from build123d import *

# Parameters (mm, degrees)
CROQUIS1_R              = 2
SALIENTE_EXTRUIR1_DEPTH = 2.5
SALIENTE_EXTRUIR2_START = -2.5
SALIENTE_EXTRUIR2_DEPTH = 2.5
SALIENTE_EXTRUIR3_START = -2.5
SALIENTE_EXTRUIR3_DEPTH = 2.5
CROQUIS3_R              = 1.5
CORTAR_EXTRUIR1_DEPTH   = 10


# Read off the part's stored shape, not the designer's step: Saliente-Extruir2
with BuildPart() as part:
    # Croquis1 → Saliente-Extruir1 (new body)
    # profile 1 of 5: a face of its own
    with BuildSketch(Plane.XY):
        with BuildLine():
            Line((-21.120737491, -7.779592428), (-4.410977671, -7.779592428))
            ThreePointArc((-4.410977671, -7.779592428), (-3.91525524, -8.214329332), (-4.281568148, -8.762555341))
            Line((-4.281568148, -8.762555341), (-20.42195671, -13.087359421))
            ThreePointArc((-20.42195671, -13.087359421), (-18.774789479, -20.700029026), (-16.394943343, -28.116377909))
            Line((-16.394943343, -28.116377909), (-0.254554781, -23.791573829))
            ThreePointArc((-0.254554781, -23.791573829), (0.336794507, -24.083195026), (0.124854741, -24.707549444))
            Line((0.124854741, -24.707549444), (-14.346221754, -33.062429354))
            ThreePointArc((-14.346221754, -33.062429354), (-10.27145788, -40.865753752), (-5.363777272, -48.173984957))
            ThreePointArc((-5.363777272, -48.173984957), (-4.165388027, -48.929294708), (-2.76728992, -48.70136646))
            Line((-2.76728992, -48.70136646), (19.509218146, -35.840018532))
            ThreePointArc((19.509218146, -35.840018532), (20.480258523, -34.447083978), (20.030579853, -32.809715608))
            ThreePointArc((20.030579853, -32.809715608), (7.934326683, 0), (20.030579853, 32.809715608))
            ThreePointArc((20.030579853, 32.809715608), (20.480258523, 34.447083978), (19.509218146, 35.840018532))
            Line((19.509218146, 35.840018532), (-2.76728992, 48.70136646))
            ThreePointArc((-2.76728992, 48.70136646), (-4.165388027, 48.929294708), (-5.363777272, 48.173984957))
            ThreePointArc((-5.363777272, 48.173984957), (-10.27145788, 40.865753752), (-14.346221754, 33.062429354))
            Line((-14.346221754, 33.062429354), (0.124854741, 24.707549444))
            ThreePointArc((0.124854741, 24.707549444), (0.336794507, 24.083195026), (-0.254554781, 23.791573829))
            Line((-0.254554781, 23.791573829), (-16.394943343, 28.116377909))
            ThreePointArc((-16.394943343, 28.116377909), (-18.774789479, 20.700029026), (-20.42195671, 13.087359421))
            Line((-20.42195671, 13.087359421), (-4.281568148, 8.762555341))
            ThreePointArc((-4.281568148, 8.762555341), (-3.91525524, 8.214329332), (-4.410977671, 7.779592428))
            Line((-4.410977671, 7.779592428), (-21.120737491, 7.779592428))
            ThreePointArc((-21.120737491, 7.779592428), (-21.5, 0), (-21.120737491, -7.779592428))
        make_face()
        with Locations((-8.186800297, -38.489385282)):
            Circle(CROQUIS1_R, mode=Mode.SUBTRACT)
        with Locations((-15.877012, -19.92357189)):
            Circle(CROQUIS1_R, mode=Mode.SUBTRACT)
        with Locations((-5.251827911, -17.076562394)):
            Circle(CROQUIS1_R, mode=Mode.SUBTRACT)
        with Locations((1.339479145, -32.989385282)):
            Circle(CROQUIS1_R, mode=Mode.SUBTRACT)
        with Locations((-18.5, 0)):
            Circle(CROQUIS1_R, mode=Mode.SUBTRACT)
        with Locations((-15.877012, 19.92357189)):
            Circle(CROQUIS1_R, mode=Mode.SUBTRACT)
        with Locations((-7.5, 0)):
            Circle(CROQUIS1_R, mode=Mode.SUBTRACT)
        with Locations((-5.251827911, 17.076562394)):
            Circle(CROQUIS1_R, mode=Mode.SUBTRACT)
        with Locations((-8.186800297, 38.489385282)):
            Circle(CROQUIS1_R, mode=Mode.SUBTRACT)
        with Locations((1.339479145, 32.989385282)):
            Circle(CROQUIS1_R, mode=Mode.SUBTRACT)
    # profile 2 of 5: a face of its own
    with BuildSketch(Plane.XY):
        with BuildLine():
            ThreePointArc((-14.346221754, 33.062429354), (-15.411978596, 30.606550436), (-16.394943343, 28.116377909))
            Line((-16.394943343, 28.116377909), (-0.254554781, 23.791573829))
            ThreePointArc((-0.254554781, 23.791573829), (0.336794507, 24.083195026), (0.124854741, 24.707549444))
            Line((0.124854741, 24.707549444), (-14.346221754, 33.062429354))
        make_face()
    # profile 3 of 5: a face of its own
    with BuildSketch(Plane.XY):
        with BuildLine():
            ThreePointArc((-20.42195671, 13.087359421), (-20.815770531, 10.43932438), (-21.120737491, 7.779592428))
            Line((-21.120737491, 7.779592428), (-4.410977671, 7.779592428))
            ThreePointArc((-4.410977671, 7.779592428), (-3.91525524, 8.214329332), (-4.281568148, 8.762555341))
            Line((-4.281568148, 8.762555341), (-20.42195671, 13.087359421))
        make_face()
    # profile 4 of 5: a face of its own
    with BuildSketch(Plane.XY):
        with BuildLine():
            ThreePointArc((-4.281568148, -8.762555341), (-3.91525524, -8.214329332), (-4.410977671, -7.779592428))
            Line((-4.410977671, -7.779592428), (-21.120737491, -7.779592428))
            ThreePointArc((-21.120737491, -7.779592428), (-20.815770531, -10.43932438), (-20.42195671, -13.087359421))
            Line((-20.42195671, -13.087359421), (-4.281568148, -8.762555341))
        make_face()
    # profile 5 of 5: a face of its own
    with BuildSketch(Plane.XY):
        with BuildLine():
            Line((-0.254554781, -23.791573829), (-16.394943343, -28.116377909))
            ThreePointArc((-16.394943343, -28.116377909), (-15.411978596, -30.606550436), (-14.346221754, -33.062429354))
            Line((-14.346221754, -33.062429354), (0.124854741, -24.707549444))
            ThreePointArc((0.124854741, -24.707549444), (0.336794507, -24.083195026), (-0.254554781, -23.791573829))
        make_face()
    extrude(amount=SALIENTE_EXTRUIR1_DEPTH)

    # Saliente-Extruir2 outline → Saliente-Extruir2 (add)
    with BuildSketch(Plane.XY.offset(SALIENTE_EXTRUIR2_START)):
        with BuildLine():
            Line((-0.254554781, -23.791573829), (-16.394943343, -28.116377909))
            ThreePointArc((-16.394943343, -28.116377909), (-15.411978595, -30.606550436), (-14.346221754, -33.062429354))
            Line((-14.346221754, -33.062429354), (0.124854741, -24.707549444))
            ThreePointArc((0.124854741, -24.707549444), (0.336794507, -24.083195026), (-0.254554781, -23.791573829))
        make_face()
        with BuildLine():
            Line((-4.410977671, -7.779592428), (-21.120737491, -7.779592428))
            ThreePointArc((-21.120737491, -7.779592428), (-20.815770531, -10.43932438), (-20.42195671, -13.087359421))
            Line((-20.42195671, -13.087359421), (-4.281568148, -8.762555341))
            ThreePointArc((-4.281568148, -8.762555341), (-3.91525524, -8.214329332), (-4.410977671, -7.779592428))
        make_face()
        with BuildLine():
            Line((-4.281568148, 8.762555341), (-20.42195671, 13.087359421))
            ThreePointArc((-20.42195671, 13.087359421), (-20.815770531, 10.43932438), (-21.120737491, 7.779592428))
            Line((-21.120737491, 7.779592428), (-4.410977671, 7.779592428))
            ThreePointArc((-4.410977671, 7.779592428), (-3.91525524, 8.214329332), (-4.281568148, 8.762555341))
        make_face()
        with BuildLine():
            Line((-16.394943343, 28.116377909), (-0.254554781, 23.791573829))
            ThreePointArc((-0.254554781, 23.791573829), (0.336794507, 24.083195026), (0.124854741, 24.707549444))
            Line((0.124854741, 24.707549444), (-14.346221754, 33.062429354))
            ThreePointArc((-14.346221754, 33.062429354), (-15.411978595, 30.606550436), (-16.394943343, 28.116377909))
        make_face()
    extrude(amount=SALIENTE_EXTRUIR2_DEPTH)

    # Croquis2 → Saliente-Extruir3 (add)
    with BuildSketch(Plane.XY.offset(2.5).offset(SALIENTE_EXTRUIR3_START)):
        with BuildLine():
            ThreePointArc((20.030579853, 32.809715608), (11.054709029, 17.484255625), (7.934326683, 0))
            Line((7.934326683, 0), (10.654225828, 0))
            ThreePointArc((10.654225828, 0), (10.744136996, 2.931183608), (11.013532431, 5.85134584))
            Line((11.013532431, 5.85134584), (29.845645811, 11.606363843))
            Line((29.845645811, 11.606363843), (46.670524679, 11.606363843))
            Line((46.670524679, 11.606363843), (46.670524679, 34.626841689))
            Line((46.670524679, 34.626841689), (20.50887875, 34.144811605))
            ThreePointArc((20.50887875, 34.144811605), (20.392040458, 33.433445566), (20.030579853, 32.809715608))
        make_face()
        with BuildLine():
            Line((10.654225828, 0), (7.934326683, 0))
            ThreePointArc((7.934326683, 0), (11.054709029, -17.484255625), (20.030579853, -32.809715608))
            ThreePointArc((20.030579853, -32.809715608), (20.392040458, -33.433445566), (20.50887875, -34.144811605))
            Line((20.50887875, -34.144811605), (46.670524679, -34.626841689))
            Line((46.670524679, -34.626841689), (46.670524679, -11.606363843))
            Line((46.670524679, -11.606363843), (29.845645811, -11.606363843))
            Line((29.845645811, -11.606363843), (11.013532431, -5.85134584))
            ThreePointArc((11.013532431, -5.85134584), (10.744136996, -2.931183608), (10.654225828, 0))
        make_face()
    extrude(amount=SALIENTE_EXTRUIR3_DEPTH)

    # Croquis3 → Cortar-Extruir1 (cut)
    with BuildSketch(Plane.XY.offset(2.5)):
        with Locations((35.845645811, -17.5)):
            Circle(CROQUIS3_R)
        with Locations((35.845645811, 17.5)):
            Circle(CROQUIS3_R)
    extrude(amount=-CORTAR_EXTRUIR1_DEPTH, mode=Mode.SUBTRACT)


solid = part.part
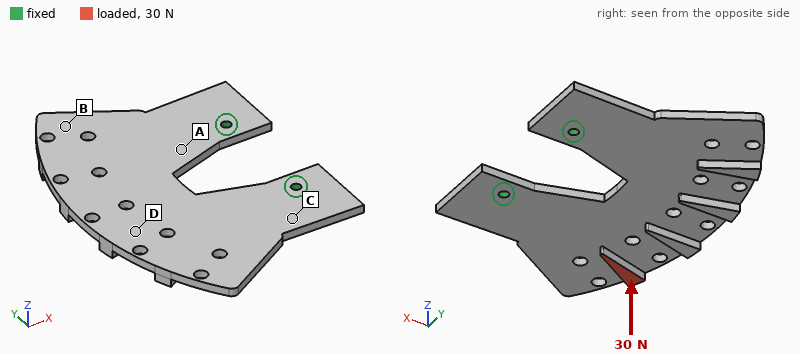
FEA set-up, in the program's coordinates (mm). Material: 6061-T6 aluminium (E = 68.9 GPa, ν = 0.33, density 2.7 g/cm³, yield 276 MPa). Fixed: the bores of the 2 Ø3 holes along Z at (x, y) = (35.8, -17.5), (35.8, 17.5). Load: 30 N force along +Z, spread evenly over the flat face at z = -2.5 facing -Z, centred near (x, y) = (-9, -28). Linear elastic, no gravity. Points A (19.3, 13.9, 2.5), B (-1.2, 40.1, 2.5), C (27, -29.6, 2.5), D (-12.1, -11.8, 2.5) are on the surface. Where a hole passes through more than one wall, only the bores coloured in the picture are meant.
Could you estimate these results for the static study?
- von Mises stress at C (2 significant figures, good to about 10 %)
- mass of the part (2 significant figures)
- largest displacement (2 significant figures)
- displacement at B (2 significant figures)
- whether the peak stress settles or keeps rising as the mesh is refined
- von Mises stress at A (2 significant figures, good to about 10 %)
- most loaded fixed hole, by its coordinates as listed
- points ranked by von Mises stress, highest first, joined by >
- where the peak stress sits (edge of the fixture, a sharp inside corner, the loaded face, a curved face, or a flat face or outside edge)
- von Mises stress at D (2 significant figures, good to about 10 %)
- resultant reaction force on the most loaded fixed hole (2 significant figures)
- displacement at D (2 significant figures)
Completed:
26 MPa
30 g
0.37 mm
0.081 mm
keeps rising
14 MPa
(35.8, -17.5)
C > A > D > B
edge of the fixture
6.9 MPa
27 N
0.28 mm
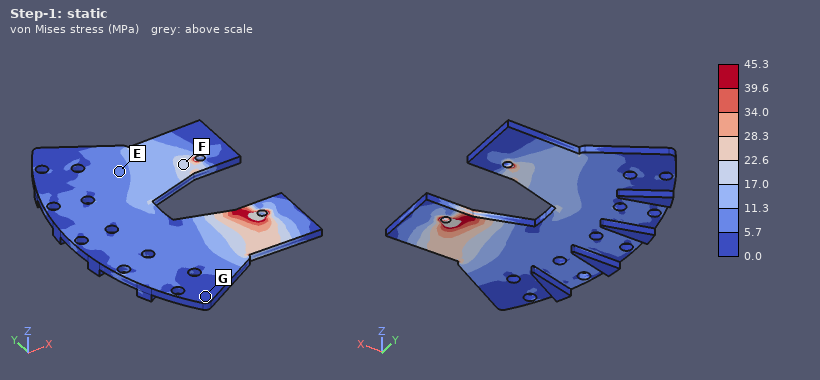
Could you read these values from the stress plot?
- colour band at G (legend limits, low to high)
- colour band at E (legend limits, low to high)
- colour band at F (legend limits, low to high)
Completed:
0.0 to 5.7 MPa
5.7 to 11.3 MPa
17.0 to 22.6 MPa
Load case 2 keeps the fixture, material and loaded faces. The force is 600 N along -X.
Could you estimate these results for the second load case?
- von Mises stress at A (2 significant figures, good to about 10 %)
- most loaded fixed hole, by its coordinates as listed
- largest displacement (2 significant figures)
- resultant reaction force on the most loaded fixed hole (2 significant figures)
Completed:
38 MPa
(35.8, -17.5)
0.82 mm
740 N
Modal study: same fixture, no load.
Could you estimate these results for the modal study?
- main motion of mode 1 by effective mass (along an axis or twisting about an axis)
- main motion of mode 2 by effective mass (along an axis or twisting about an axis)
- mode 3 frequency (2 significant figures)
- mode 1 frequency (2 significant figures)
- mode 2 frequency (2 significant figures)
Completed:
along Z
twisting about X
2000 Hz
490 Hz
940 Hz
